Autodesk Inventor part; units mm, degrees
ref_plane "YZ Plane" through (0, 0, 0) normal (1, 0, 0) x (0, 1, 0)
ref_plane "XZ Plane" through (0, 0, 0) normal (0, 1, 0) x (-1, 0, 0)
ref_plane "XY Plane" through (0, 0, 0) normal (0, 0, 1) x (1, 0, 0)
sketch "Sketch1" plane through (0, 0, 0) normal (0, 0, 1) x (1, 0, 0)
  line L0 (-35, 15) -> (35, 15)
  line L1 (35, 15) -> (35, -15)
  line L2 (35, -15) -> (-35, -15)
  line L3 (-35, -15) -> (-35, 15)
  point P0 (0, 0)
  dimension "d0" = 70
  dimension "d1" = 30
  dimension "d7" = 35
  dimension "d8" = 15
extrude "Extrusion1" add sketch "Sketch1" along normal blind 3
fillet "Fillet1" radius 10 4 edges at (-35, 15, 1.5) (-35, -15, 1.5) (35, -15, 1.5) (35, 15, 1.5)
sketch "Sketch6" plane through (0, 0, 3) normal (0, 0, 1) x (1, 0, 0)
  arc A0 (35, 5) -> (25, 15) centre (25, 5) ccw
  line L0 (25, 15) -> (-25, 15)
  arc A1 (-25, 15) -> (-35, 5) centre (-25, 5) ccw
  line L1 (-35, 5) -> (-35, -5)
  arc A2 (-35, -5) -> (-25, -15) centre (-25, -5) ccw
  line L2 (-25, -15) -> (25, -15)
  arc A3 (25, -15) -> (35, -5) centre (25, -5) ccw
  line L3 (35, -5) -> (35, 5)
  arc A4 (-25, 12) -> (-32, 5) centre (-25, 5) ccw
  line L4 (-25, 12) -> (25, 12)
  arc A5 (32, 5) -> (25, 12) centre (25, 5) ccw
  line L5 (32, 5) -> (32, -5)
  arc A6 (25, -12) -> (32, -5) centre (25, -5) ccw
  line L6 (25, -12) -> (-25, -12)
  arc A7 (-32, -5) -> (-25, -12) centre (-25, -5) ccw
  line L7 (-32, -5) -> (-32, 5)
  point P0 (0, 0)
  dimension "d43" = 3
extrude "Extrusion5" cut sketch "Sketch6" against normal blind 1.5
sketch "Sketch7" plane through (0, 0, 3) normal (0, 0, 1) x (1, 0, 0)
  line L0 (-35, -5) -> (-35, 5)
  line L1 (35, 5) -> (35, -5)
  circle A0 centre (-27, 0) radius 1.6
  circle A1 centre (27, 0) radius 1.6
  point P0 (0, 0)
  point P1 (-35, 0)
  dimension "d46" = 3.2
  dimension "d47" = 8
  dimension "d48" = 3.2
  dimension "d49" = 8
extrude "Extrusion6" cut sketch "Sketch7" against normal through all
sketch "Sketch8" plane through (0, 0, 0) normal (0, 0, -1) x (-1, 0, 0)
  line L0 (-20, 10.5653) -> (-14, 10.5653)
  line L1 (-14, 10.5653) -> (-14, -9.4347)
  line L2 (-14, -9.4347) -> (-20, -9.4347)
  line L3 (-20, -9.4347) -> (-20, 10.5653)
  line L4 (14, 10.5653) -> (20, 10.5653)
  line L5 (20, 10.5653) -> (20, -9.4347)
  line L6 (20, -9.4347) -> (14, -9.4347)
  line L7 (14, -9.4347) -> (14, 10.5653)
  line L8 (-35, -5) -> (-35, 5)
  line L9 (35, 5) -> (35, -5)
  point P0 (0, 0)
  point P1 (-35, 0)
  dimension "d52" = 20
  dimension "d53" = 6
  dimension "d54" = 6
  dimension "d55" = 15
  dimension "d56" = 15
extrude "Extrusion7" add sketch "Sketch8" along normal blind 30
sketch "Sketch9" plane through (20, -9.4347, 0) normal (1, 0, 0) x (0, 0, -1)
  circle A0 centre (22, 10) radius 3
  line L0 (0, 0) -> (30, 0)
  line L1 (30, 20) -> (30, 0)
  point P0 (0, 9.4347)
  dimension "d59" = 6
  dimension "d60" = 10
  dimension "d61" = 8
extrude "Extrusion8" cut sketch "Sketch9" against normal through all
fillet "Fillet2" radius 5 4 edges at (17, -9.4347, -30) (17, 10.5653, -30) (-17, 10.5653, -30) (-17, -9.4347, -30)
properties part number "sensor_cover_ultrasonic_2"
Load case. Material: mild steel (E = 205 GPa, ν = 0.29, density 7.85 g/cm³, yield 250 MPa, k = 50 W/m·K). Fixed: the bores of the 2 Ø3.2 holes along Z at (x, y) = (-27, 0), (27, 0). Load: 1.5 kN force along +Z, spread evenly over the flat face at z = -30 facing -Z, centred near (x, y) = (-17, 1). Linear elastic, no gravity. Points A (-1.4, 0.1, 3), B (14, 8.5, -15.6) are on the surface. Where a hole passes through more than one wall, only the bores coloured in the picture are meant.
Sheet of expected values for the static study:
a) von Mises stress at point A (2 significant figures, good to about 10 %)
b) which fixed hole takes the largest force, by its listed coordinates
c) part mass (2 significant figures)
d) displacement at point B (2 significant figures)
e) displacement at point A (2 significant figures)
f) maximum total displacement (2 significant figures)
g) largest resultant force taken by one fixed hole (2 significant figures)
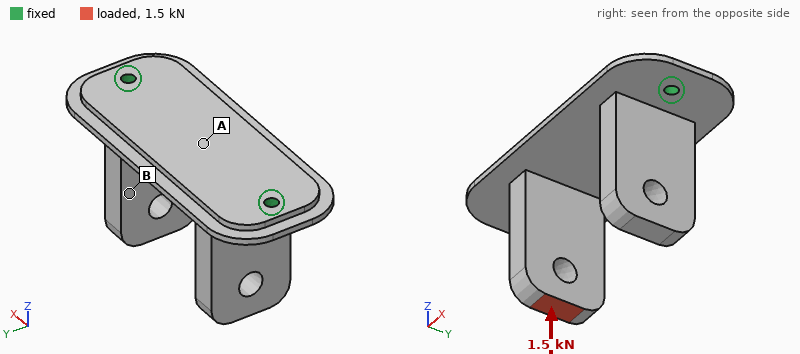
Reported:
49 MPa
(-27, 0)
94 g
0.037 mm
0.044 mm
0.10 mm
1.3 kN
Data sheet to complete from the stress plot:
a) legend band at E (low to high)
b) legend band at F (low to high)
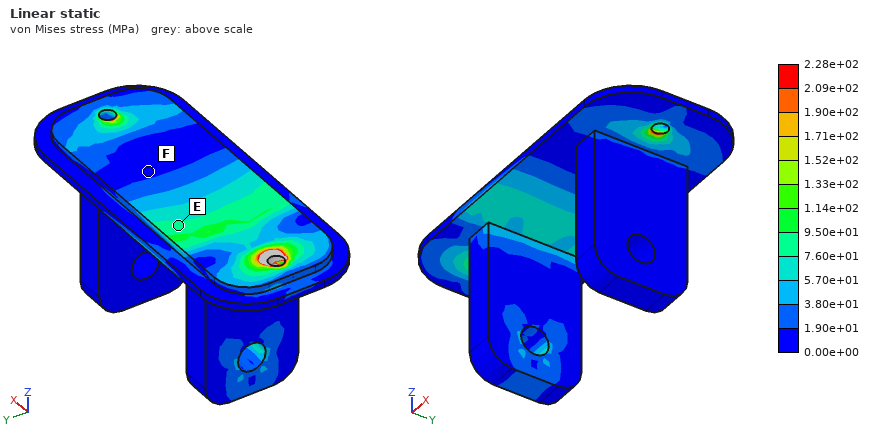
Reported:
7.60e+01 to 9.50e+01 MPa
0.00e+00 to 1.90e+01 MPa
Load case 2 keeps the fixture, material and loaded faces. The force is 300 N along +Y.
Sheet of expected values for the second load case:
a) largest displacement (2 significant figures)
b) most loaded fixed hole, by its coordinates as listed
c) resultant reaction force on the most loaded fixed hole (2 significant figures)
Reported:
0.11 mm
(-27, 0)
250 N
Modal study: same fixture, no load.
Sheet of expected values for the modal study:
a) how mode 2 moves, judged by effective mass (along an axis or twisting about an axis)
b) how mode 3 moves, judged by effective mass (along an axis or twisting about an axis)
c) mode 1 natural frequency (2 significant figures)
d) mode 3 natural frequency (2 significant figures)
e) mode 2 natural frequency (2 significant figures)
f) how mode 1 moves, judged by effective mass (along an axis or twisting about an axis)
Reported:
along Y
twisting about Z
2000 Hz
3100 Hz
2300 Hz
along Z
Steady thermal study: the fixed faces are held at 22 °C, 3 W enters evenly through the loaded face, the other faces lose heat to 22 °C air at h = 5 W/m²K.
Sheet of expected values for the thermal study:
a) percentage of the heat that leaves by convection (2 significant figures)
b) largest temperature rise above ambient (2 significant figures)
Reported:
7.1 %
26 K
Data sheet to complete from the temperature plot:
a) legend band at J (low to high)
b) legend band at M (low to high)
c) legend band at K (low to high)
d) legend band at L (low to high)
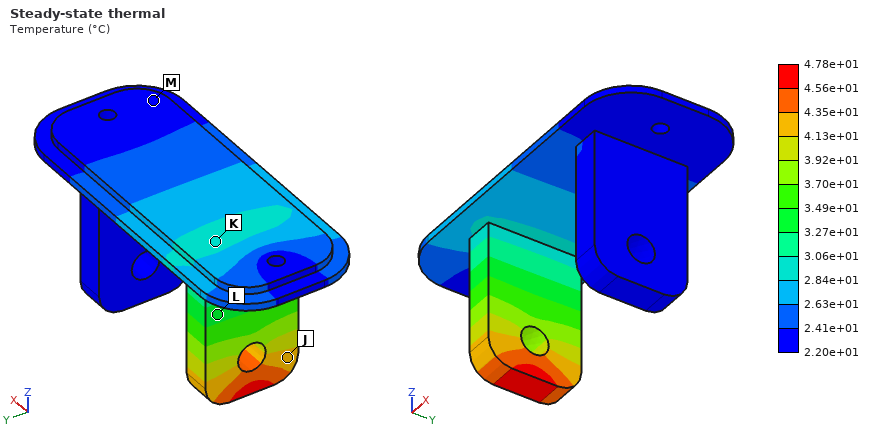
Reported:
4.13e+01 to 4.35e+01 °C
2.20e+01 to 2.41e+01 °C
2.84e+01 to 3.06e+01 °C
3.27e+01 to 3.49e+01 °C
